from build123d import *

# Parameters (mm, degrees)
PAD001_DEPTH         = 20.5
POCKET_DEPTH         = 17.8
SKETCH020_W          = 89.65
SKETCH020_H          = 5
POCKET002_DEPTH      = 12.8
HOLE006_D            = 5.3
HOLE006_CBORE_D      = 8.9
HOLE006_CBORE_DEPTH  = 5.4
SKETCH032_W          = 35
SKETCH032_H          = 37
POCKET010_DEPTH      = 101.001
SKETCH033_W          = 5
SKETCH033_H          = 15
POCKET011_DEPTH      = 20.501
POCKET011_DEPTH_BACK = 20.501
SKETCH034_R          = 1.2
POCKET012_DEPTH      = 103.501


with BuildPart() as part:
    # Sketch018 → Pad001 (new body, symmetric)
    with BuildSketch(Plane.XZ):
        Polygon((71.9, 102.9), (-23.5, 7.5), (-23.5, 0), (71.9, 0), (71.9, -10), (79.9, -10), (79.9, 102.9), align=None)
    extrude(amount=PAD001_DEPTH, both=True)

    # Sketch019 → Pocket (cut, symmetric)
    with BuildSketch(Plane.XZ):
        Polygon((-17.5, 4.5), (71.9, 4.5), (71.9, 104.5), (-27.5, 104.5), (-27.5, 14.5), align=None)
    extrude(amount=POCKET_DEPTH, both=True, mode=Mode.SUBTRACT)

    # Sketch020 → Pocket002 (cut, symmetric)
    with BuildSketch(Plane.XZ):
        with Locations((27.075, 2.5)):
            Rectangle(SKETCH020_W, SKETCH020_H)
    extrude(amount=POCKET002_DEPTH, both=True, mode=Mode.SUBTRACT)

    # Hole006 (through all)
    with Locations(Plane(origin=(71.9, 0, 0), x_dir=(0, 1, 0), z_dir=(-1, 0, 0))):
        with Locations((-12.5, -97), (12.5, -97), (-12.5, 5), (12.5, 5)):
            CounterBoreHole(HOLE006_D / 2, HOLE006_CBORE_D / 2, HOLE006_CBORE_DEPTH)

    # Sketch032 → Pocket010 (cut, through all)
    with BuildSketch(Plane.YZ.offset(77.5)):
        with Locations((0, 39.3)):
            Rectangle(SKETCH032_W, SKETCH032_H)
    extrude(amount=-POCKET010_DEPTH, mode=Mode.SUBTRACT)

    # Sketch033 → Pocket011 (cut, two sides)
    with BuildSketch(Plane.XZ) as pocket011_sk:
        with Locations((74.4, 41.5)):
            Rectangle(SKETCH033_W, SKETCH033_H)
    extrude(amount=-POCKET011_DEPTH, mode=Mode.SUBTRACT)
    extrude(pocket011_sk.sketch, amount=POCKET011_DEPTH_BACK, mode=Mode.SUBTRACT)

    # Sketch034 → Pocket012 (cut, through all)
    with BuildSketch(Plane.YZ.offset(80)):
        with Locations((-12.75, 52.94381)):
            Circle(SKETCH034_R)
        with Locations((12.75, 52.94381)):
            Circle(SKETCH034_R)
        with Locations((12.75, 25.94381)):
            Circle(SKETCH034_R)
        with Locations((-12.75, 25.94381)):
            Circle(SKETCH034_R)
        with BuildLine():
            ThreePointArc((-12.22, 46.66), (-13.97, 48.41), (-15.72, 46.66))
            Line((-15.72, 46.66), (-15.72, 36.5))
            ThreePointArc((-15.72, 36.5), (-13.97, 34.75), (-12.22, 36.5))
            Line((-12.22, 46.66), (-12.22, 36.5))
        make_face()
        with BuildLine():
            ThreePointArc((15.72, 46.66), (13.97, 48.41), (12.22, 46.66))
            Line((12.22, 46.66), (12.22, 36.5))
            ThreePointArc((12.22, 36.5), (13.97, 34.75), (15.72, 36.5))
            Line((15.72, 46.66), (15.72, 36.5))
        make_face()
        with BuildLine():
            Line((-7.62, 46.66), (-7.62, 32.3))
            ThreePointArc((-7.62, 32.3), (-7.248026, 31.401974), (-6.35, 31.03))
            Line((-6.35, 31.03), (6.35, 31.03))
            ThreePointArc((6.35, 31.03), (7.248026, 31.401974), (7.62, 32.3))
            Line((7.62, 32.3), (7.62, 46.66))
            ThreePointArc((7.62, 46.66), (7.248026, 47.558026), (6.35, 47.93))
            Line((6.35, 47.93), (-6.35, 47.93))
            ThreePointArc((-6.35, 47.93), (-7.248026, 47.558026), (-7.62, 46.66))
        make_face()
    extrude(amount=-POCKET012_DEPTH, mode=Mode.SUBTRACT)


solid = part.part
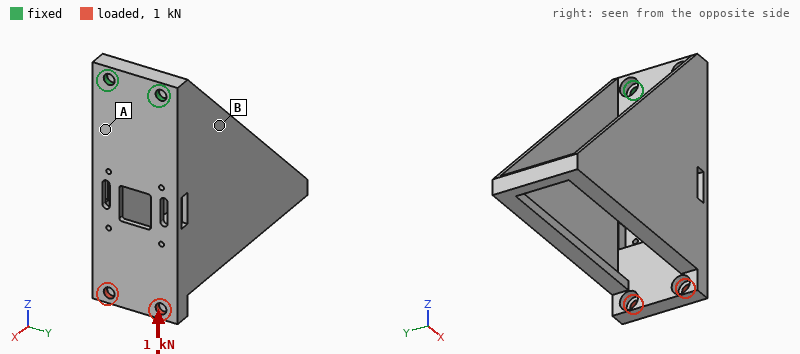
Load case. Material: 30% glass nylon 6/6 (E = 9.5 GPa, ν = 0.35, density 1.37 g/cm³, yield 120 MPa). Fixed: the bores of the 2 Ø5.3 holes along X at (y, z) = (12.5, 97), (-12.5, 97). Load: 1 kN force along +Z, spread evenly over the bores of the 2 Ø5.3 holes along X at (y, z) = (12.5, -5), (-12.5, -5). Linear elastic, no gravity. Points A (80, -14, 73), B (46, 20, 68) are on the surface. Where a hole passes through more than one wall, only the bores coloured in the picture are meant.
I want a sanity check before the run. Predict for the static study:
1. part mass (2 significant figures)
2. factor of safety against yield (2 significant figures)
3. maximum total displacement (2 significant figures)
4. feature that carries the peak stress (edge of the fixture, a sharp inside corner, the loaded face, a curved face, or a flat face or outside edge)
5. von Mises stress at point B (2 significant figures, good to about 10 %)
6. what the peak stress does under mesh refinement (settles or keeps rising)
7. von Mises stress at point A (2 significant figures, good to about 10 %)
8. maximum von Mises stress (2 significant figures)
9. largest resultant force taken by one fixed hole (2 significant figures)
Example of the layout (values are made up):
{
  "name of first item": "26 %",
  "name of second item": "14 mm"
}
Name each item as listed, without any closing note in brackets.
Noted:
{
  "part mass": "83 g",
  "factor of safety against yield": "3.6",
  "maximum total displacement": "0.26 mm",
  "feature that carries the peak stress": "the loaded face",
  "von Mises stress at point B": "2.4 MPa",
  "what the peak stress does under mesh refinement": "settles",
  "von Mises stress at point A": "5.5 MPa",
  "maximum von Mises stress": "33 MPa",
  "largest resultant force taken by one fixed hole": "500 N"
}
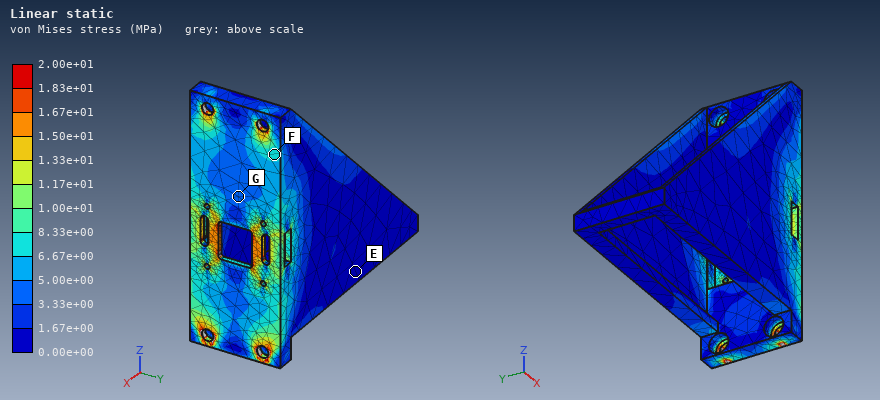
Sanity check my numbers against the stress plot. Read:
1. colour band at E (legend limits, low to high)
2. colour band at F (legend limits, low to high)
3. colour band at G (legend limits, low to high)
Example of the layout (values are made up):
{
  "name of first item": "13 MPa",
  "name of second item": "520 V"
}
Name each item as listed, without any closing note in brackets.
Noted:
{
  "colour band at E": "0.00e+00 to 1.67e+00 MPa",
  "colour band at F": "6.67e+00 to 8.33e+00 MPa",
  "colour band at G": "3.33e+00 to 5.00e+00 MPa"
}
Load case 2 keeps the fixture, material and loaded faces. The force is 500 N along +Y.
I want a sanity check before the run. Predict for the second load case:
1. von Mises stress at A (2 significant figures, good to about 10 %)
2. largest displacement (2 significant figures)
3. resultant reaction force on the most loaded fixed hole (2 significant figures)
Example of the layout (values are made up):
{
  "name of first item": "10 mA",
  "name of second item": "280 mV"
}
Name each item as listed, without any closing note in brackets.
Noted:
{
  "von Mises stress at A": "13 MPa",
  "largest displacement": "1.1 mm",
  "resultant reaction force on the most loaded fixed hole": "1.8 kN"
}
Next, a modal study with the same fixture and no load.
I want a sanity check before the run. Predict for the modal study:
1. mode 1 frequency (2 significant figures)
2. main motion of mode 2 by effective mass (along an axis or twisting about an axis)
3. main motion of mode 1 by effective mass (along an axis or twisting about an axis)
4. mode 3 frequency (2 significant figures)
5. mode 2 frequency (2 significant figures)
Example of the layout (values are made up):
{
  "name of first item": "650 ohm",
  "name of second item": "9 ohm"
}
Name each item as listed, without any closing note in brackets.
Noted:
{
  "mode 1 frequency": "170 Hz",
  "main motion of mode 2 by effective mass": "along Y",
  "main motion of mode 1 by effective mass": "along X",
  "mode 3 frequency": "690 Hz",
  "mode 2 frequency": "190 Hz"
}
